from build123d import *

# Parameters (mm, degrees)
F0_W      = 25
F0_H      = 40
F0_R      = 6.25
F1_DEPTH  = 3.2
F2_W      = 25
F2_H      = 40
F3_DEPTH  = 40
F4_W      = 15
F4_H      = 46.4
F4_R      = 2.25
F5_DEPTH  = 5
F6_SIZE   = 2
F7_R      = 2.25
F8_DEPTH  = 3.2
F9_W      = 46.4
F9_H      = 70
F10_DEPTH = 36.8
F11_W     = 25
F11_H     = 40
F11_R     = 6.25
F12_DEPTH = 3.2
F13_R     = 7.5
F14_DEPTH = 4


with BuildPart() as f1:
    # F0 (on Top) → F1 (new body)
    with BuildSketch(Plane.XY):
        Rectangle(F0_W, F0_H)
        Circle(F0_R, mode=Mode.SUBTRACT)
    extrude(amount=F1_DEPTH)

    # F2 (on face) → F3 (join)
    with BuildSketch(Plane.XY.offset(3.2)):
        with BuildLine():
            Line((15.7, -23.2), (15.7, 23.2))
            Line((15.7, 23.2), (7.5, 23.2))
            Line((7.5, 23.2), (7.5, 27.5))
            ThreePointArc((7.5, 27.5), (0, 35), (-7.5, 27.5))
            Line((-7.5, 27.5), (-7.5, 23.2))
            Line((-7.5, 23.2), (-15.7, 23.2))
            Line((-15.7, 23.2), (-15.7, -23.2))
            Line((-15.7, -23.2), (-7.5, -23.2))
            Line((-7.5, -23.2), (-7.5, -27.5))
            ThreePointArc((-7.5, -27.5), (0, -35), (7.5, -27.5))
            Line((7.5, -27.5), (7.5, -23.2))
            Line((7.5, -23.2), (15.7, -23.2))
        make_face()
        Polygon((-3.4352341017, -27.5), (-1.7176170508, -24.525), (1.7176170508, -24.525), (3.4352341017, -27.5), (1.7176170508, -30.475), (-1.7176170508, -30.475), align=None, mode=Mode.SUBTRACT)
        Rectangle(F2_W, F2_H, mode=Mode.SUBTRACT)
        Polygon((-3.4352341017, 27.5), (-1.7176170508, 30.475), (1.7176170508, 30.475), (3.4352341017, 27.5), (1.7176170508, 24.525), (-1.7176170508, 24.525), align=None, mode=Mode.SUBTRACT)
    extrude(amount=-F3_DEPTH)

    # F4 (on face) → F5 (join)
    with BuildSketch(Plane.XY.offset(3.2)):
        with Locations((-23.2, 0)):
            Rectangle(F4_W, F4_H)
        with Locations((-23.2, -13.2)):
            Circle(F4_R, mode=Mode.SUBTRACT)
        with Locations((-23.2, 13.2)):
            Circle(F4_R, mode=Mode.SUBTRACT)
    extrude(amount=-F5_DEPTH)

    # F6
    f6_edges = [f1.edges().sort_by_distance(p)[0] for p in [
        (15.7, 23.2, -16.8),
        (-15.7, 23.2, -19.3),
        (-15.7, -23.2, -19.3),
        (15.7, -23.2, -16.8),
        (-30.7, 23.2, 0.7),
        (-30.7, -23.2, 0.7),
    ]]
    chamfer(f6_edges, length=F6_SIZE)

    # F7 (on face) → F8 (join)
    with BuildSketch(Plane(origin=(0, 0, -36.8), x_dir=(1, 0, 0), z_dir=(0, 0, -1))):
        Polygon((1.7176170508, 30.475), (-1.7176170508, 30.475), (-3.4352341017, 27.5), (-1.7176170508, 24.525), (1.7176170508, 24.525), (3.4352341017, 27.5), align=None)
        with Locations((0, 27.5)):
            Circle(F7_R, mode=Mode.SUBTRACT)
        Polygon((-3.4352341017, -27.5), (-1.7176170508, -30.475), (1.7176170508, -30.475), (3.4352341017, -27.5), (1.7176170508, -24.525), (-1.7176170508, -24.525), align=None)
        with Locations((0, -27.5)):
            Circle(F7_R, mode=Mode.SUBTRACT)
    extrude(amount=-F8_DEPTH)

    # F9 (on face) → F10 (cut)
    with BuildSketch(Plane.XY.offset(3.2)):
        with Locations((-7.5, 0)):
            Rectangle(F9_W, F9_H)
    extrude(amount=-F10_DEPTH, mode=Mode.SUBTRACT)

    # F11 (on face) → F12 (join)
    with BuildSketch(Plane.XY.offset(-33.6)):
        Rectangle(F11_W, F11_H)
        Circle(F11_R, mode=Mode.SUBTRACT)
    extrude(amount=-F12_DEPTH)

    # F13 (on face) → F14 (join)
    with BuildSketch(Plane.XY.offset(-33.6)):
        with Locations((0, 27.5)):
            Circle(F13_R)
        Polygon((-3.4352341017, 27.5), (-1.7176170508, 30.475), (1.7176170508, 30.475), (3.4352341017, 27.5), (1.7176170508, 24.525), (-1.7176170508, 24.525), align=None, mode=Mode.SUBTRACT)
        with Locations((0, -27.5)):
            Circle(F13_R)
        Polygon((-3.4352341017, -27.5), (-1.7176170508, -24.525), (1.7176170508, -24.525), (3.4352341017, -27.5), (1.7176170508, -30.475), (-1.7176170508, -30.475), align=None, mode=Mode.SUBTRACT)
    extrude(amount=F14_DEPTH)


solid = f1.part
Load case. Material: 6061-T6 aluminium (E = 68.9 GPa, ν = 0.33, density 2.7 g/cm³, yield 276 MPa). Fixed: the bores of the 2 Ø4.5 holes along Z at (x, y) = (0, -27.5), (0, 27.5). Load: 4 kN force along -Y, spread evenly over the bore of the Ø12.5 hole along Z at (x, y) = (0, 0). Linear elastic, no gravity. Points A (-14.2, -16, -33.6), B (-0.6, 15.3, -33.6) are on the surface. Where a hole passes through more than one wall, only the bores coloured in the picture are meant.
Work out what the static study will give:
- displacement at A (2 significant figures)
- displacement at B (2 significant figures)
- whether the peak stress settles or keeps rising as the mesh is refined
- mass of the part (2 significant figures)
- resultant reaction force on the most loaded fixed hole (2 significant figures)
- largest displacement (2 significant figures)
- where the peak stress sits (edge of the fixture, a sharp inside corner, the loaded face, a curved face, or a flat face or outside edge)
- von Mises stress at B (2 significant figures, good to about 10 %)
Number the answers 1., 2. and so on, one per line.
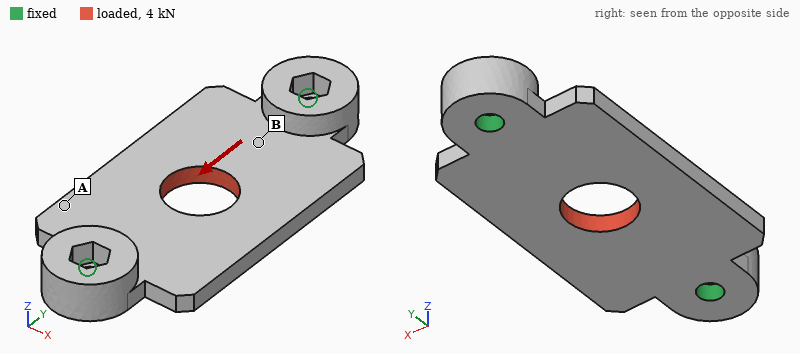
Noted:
1. 8.8 µm
2. 6.6 µm
3. keeps rising
4. 17 g
5. 2.0 kN
6. 14 µm
7. edge of the fixture
8. 43 MPa
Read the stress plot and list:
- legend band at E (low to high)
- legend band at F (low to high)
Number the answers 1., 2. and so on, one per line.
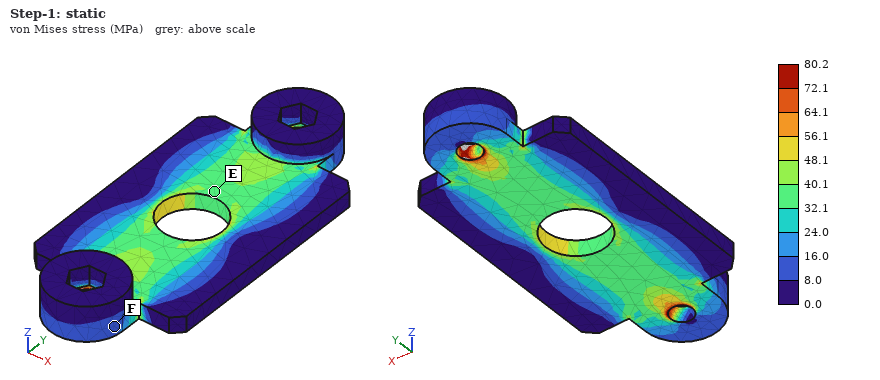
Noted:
1. 32.1 to 40.1 MPa
2. 8.0 to 16.0 MPa
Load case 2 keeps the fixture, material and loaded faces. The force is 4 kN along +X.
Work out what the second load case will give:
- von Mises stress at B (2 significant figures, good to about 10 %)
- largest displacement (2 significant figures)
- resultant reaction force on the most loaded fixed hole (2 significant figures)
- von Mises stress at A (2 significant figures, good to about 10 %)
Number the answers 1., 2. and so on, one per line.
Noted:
1. 41 MPa
2. 44 µm
3. 2.0 kN
4. 26 MPa
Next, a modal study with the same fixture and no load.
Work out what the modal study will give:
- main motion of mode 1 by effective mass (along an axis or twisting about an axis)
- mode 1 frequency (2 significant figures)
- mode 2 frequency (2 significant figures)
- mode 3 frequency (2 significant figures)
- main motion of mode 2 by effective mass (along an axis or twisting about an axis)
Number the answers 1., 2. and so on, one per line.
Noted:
1. along Z
2. 5400 Hz
3. 5800 Hz
4. 12 kHz
5. twisting about Y
